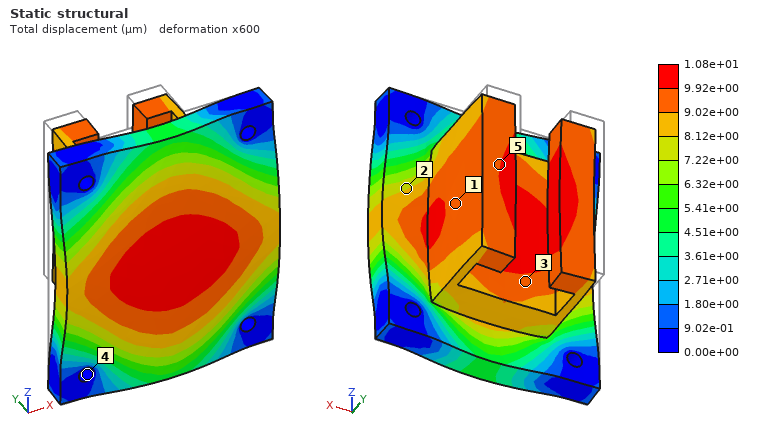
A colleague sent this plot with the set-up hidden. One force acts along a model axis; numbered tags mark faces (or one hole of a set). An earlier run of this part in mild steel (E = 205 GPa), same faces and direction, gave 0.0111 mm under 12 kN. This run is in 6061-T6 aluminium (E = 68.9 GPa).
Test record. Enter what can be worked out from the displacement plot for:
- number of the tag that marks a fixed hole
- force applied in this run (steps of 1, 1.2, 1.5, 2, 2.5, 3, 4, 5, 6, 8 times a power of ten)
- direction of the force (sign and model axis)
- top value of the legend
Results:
4
4 kN
-Y
1.08e+01 µm
